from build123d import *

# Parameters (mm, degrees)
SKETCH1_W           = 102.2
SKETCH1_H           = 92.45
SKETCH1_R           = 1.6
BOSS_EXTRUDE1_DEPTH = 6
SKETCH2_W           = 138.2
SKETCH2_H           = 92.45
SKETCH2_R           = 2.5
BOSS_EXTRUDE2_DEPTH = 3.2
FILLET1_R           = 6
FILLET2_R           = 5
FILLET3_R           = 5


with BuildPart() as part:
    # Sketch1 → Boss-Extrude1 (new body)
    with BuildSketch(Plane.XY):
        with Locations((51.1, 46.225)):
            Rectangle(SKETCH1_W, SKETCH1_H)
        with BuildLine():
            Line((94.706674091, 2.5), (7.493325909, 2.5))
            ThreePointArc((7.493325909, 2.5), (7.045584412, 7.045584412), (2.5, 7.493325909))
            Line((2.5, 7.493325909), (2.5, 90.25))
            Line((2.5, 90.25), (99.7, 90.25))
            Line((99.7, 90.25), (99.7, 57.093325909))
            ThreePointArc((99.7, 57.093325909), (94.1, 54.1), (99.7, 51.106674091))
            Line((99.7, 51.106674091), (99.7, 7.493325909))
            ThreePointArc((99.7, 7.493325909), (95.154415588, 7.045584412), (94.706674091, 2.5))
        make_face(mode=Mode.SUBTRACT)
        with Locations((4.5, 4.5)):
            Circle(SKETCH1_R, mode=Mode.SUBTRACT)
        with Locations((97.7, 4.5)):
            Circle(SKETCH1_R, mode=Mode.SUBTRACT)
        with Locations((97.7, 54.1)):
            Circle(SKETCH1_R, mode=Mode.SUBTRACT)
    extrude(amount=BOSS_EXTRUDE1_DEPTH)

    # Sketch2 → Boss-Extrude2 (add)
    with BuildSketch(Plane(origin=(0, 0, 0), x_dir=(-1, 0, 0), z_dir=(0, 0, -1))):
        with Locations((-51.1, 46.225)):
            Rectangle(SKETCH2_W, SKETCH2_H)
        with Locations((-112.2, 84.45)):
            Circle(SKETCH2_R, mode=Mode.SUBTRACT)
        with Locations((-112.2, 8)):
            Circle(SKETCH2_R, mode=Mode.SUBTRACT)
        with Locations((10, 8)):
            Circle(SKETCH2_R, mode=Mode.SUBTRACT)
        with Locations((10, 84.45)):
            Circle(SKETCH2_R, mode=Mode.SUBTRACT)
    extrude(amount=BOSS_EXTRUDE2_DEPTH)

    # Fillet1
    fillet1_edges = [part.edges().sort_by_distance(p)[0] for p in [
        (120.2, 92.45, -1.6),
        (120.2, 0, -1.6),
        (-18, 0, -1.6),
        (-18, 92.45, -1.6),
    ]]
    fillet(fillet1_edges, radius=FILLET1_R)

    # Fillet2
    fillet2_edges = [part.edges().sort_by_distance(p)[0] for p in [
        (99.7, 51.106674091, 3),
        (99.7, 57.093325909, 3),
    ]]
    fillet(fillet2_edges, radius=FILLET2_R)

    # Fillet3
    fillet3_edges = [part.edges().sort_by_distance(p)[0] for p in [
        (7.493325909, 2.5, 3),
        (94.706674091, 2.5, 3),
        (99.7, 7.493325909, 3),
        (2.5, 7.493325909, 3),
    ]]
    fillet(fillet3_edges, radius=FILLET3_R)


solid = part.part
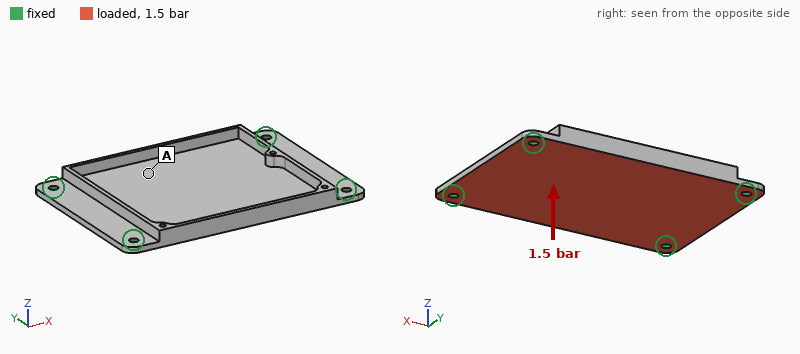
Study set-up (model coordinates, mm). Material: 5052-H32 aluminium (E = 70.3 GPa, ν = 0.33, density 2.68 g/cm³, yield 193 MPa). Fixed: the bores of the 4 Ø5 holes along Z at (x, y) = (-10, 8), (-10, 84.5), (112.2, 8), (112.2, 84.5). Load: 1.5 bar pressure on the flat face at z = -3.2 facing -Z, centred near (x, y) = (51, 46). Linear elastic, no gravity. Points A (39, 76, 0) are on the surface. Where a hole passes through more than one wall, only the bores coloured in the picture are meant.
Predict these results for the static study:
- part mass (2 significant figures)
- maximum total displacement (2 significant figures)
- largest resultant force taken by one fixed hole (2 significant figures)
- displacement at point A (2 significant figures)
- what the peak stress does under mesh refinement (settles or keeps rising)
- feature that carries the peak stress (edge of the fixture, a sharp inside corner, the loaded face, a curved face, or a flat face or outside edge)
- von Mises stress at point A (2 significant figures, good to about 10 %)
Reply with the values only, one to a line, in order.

120 g
0.39 mm
620 N
0.30 mm
keeps rising
edge of the fixture
27 MPa
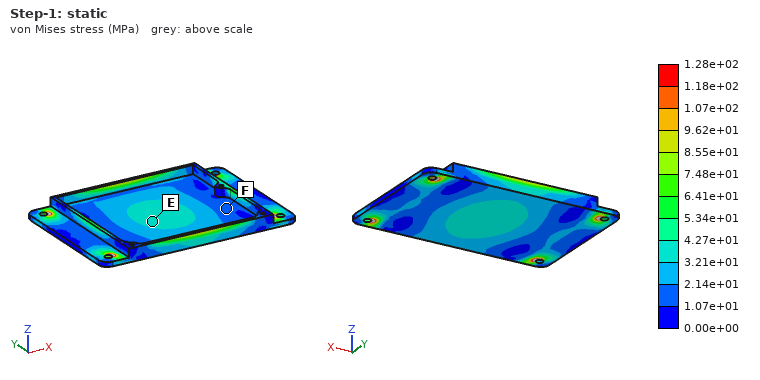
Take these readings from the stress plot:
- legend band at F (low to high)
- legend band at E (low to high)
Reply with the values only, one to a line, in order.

1.07e+01 to 2.14e+01 MPa
3.21e+01 to 4.27e+01 MPa
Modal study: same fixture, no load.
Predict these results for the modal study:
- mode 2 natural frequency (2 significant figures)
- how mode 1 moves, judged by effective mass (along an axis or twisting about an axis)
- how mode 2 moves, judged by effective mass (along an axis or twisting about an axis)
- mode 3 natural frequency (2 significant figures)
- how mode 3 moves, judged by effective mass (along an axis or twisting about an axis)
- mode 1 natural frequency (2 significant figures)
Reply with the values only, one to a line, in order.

2000 Hz
along Z
twisting about X
2900 Hz
twisting about Y
1200 Hz
